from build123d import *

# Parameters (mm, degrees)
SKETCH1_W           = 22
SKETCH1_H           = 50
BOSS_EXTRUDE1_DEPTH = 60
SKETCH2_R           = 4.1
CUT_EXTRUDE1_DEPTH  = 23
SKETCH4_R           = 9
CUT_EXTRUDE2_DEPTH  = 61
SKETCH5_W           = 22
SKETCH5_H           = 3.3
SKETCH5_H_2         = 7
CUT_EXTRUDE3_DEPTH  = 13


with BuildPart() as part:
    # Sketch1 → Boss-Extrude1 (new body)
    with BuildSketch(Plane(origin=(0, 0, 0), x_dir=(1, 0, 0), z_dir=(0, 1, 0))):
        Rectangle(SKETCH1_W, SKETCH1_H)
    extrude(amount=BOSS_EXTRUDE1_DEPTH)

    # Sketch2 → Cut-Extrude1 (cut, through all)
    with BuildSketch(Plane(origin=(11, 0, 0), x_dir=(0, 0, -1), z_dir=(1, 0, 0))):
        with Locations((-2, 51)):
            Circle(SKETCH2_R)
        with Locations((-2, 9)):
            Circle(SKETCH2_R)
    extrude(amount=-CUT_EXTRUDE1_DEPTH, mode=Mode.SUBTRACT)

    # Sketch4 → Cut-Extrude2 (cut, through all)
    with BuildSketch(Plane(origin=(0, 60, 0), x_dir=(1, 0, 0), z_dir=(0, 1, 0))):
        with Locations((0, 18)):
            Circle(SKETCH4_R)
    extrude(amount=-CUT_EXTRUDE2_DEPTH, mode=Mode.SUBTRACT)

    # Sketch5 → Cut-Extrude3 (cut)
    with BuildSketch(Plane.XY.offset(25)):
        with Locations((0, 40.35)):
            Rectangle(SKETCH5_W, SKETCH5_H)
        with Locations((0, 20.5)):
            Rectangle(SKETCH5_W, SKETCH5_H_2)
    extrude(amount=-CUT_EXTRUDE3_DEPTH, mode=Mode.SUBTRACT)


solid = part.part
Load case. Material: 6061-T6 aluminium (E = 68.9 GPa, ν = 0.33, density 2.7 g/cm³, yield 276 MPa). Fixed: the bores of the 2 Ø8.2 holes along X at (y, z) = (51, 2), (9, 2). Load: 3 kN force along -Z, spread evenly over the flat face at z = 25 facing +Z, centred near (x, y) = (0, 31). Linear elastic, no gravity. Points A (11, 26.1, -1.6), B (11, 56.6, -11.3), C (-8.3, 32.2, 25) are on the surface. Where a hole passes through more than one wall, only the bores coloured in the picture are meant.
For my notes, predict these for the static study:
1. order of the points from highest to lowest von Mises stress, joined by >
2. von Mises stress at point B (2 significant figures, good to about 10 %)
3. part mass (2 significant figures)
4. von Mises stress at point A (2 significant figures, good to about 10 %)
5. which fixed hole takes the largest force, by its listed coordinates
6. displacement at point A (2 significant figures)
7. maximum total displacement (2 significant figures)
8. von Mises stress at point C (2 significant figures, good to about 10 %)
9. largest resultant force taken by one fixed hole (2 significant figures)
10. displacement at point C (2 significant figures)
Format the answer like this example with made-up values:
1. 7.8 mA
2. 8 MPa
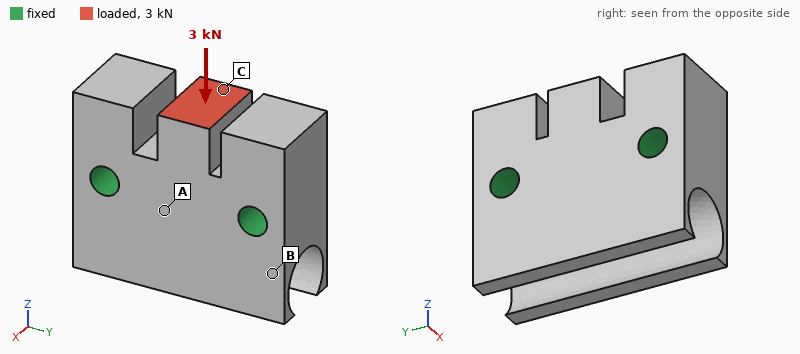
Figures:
1. C > A > B
2. 1.6 MPa
3. 130 g
4. 4.3 MPa
5. (51, 2)
6. 1.9 µm
7. 4.6 µm
8. 9.4 MPa
9. 1.6 kN
10. 4.4 µm
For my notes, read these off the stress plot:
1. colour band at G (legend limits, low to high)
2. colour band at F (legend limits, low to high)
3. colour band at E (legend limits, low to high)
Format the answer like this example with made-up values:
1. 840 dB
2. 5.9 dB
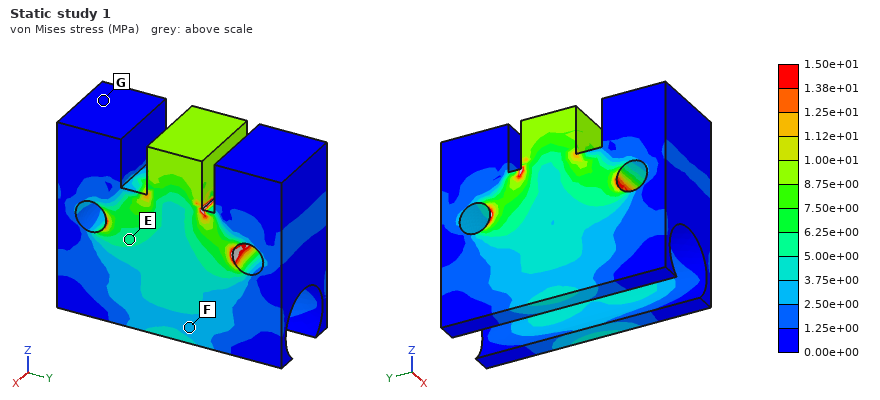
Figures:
1. 0.00e+00 to 1.25e+00 MPa
2. 2.50e+00 to 3.75e+00 MPa
3. 5.00e+00 to 6.25e+00 MPa
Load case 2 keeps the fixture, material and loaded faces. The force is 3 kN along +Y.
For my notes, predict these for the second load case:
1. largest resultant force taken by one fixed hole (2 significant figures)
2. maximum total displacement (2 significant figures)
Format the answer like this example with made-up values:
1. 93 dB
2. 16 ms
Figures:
1. 2.4 kN
2. 23 µm
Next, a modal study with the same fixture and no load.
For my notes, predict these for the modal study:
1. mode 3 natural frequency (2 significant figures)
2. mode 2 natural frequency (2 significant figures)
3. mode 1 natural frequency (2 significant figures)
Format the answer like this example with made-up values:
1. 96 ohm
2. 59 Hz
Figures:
1. 11 kHz
2. 9500 Hz
3. 9300 Hz
